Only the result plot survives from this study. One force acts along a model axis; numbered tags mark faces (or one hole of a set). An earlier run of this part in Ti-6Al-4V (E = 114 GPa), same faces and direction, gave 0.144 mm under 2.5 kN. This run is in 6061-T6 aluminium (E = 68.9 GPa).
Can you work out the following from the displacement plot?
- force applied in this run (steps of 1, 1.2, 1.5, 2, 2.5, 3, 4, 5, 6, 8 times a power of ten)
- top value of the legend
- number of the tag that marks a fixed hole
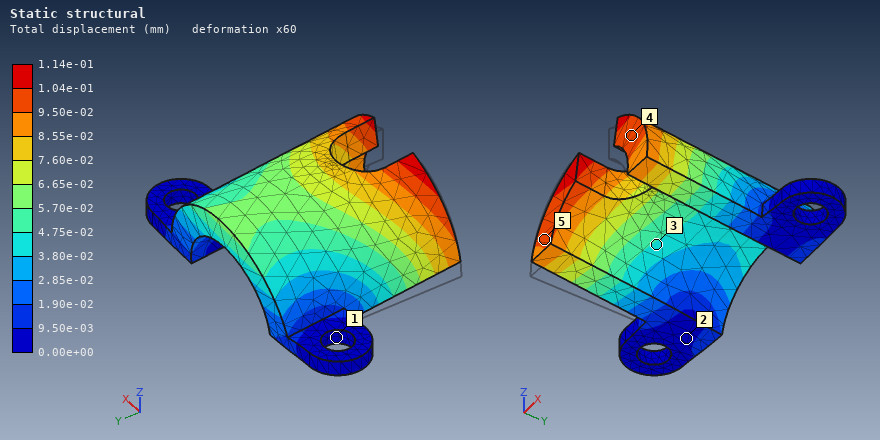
1.2 kN
1.14e-01 mm
1
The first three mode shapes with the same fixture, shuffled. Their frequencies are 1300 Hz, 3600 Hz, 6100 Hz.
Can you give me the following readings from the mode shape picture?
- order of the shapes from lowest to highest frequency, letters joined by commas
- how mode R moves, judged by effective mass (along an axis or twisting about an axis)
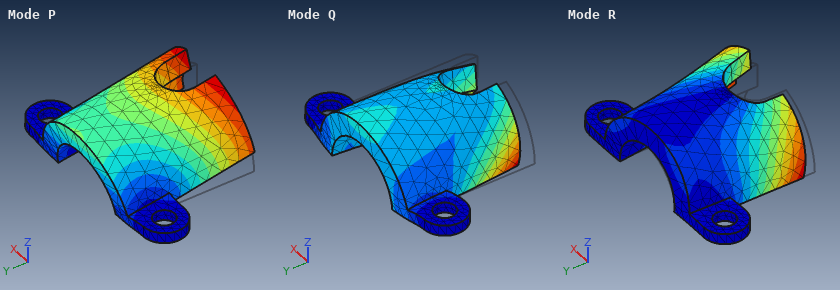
P, R, Q
along X
